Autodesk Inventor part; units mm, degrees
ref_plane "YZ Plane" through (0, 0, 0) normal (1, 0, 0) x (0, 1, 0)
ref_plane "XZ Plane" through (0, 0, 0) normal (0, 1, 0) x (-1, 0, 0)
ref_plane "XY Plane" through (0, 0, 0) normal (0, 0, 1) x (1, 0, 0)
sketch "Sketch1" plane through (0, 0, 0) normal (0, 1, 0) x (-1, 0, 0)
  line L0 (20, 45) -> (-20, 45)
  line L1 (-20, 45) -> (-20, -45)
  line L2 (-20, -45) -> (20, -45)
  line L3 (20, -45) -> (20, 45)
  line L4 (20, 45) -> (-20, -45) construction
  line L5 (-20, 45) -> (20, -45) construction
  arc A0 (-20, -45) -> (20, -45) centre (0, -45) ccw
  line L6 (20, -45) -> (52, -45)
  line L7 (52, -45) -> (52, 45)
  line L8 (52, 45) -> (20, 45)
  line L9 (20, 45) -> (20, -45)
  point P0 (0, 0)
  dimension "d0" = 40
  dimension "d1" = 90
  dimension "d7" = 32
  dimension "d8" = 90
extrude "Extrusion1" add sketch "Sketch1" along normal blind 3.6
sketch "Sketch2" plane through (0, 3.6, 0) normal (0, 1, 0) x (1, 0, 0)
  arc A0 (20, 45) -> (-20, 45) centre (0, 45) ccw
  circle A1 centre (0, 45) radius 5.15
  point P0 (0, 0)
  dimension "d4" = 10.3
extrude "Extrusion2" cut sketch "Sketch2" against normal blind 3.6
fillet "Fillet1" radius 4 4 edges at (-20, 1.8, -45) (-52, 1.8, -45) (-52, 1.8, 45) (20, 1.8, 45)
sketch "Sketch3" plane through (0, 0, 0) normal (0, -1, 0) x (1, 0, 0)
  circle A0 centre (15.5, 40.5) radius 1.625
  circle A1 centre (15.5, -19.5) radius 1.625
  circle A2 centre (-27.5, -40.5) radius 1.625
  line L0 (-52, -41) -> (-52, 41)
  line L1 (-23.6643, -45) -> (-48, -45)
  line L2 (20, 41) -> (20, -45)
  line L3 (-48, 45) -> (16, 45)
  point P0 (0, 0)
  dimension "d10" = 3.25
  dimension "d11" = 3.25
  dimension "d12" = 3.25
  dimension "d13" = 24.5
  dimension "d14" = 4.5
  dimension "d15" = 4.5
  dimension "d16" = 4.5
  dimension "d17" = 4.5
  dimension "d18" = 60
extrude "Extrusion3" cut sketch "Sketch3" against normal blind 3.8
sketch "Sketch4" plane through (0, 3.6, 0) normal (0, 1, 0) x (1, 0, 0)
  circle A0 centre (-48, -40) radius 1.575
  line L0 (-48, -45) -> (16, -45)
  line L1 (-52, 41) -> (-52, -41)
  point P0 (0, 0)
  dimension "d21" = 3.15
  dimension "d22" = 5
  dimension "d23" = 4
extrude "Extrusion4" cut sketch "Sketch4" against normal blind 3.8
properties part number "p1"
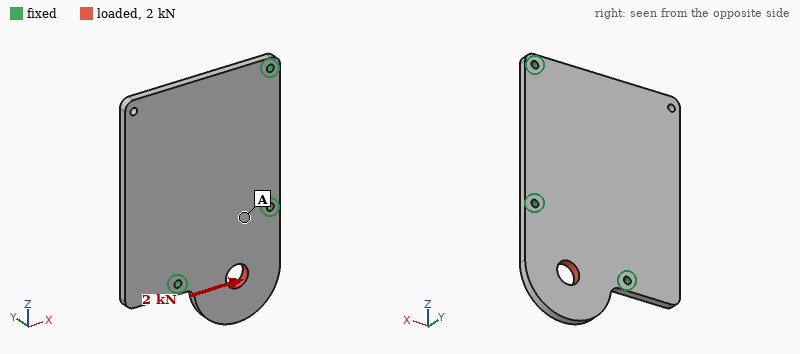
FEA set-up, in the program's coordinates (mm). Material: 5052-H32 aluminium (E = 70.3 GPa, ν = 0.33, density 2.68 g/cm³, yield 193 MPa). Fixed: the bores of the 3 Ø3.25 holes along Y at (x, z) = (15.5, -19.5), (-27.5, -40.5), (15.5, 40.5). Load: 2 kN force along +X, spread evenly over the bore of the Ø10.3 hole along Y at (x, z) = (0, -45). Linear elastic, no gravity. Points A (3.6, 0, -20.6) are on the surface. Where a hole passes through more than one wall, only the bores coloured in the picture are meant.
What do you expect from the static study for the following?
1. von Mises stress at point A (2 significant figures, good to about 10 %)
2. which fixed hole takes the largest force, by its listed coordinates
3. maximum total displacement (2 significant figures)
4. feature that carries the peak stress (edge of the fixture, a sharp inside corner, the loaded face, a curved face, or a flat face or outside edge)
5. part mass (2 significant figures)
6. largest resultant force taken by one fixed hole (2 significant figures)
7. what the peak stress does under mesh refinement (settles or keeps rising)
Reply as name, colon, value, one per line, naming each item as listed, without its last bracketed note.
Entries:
von Mises stress at point A: 6.9 MPa
which fixed hole takes the largest force, by its listed coordinates: (-27.5, -40.5)
maximum total displacement: 16 µm
feature that carries the peak stress: edge of the fixture
part mass: 67 g
largest resultant force taken by one fixed hole: 1.4 kN
what the peak stress does under mesh refinement: keeps rising
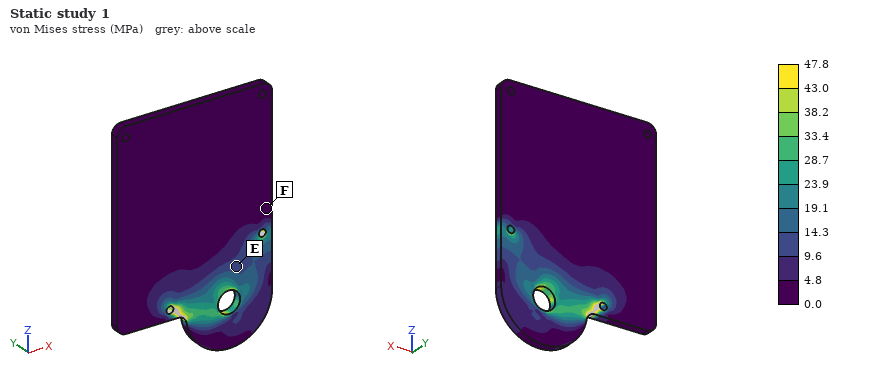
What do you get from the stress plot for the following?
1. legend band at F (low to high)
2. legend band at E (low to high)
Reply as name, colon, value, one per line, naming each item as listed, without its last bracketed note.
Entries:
legend band at F: 0.0 to 4.8 MPa
legend band at E: 9.6 to 14.3 MPa
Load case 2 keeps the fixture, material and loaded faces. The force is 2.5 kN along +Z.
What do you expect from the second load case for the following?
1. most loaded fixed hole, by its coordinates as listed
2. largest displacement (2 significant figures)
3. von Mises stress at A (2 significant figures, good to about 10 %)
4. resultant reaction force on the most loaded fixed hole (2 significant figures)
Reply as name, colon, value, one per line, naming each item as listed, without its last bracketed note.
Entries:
most loaded fixed hole, by its coordinates as listed: (15.5, -19.5)
largest displacement: 13 µm
von Mises stress at A: 12 MPa
resultant reaction force on the most loaded fixed hole: 1.5 kN
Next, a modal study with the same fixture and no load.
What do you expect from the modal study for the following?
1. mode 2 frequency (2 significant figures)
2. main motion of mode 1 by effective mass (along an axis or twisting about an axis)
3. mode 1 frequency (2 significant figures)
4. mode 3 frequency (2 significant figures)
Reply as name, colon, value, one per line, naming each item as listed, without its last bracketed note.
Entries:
mode 2 frequency: 2200 Hz
main motion of mode 1 by effective mass: along Y
mode 1 frequency: 890 Hz
mode 3 frequency: 2800 Hz
